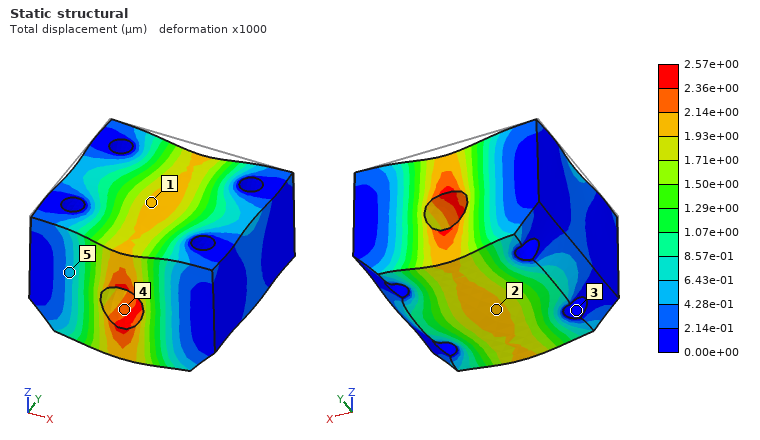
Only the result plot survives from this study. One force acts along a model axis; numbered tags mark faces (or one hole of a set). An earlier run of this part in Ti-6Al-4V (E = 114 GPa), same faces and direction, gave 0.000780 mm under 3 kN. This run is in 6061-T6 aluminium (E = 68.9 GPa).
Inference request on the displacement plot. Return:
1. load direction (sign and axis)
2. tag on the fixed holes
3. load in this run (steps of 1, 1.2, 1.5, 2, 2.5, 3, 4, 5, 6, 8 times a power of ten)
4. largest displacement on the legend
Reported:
-Z
3
6 kN
2.57e+00 µm
